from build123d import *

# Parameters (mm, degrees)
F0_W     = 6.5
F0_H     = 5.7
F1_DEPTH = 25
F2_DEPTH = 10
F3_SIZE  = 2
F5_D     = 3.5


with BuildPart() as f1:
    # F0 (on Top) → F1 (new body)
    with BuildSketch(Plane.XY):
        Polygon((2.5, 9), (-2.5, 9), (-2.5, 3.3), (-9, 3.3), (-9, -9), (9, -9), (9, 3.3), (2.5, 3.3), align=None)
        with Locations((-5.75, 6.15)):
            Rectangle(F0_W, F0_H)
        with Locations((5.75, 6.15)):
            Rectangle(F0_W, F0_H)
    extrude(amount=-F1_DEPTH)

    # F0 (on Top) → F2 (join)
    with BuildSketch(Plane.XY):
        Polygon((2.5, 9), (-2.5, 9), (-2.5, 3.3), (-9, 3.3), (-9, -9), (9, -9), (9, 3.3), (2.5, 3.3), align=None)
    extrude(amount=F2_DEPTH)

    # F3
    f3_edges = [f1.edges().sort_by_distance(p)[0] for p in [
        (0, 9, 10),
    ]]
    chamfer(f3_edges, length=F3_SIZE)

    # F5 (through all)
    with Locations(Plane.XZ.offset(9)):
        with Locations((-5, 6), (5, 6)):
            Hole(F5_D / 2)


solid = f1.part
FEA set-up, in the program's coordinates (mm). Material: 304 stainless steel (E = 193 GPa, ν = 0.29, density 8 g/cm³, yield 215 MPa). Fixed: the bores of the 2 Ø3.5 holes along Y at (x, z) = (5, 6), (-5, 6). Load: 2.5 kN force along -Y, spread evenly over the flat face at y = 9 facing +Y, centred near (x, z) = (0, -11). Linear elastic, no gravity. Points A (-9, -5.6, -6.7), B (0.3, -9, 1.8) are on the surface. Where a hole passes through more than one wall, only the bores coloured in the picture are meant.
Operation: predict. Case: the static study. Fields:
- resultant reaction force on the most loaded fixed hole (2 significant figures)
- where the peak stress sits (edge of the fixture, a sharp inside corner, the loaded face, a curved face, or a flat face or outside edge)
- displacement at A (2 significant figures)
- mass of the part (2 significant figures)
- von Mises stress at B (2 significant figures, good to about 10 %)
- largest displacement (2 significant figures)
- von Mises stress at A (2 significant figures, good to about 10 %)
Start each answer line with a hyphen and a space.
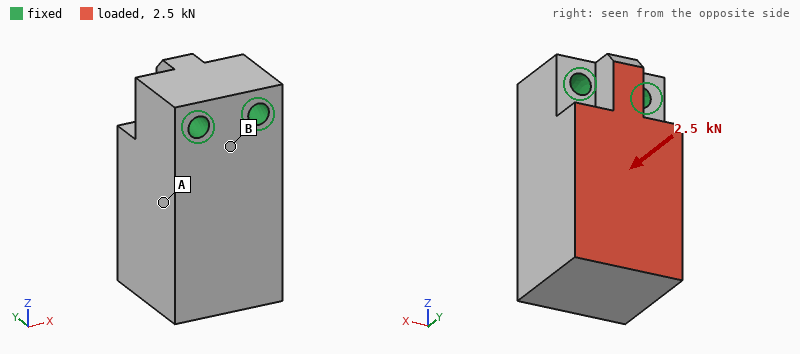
- 1.3 kN
- edge of the fixture
- 5.7 µm
- 83 g
- 43 MPa
- 18 µm
- 20 MPa
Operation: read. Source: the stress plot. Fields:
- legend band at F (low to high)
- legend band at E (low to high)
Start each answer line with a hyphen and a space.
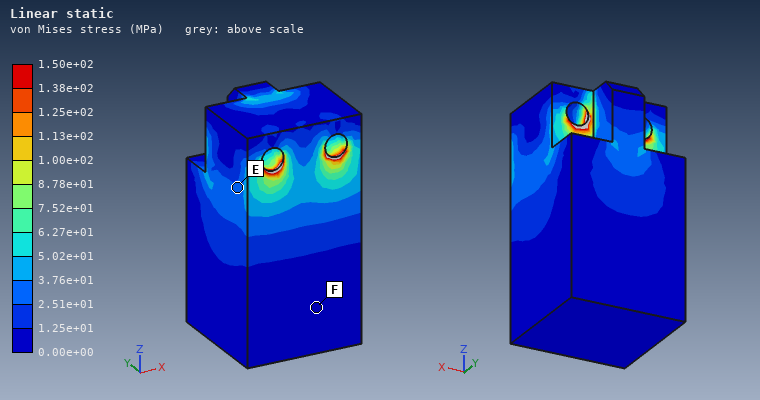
- 0.00e+00 to 1.25e+01 MPa
- 2.51e+01 to 3.76e+01 MPa
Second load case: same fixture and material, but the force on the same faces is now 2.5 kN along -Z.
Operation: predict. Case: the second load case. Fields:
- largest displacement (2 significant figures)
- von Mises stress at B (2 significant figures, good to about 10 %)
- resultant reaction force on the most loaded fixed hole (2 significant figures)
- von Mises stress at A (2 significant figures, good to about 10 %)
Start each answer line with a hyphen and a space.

- 14 µm
- 28 MPa
- 1.3 kN
- 12 MPa
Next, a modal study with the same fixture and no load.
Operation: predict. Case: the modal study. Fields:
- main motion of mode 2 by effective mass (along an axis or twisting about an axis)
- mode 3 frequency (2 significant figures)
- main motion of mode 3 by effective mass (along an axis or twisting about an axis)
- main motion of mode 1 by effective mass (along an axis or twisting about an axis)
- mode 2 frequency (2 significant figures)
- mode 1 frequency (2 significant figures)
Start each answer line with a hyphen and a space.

- along X
- 20 kHz
- twisting about Z
- along Y
- 11 kHz
- 8600 Hz
